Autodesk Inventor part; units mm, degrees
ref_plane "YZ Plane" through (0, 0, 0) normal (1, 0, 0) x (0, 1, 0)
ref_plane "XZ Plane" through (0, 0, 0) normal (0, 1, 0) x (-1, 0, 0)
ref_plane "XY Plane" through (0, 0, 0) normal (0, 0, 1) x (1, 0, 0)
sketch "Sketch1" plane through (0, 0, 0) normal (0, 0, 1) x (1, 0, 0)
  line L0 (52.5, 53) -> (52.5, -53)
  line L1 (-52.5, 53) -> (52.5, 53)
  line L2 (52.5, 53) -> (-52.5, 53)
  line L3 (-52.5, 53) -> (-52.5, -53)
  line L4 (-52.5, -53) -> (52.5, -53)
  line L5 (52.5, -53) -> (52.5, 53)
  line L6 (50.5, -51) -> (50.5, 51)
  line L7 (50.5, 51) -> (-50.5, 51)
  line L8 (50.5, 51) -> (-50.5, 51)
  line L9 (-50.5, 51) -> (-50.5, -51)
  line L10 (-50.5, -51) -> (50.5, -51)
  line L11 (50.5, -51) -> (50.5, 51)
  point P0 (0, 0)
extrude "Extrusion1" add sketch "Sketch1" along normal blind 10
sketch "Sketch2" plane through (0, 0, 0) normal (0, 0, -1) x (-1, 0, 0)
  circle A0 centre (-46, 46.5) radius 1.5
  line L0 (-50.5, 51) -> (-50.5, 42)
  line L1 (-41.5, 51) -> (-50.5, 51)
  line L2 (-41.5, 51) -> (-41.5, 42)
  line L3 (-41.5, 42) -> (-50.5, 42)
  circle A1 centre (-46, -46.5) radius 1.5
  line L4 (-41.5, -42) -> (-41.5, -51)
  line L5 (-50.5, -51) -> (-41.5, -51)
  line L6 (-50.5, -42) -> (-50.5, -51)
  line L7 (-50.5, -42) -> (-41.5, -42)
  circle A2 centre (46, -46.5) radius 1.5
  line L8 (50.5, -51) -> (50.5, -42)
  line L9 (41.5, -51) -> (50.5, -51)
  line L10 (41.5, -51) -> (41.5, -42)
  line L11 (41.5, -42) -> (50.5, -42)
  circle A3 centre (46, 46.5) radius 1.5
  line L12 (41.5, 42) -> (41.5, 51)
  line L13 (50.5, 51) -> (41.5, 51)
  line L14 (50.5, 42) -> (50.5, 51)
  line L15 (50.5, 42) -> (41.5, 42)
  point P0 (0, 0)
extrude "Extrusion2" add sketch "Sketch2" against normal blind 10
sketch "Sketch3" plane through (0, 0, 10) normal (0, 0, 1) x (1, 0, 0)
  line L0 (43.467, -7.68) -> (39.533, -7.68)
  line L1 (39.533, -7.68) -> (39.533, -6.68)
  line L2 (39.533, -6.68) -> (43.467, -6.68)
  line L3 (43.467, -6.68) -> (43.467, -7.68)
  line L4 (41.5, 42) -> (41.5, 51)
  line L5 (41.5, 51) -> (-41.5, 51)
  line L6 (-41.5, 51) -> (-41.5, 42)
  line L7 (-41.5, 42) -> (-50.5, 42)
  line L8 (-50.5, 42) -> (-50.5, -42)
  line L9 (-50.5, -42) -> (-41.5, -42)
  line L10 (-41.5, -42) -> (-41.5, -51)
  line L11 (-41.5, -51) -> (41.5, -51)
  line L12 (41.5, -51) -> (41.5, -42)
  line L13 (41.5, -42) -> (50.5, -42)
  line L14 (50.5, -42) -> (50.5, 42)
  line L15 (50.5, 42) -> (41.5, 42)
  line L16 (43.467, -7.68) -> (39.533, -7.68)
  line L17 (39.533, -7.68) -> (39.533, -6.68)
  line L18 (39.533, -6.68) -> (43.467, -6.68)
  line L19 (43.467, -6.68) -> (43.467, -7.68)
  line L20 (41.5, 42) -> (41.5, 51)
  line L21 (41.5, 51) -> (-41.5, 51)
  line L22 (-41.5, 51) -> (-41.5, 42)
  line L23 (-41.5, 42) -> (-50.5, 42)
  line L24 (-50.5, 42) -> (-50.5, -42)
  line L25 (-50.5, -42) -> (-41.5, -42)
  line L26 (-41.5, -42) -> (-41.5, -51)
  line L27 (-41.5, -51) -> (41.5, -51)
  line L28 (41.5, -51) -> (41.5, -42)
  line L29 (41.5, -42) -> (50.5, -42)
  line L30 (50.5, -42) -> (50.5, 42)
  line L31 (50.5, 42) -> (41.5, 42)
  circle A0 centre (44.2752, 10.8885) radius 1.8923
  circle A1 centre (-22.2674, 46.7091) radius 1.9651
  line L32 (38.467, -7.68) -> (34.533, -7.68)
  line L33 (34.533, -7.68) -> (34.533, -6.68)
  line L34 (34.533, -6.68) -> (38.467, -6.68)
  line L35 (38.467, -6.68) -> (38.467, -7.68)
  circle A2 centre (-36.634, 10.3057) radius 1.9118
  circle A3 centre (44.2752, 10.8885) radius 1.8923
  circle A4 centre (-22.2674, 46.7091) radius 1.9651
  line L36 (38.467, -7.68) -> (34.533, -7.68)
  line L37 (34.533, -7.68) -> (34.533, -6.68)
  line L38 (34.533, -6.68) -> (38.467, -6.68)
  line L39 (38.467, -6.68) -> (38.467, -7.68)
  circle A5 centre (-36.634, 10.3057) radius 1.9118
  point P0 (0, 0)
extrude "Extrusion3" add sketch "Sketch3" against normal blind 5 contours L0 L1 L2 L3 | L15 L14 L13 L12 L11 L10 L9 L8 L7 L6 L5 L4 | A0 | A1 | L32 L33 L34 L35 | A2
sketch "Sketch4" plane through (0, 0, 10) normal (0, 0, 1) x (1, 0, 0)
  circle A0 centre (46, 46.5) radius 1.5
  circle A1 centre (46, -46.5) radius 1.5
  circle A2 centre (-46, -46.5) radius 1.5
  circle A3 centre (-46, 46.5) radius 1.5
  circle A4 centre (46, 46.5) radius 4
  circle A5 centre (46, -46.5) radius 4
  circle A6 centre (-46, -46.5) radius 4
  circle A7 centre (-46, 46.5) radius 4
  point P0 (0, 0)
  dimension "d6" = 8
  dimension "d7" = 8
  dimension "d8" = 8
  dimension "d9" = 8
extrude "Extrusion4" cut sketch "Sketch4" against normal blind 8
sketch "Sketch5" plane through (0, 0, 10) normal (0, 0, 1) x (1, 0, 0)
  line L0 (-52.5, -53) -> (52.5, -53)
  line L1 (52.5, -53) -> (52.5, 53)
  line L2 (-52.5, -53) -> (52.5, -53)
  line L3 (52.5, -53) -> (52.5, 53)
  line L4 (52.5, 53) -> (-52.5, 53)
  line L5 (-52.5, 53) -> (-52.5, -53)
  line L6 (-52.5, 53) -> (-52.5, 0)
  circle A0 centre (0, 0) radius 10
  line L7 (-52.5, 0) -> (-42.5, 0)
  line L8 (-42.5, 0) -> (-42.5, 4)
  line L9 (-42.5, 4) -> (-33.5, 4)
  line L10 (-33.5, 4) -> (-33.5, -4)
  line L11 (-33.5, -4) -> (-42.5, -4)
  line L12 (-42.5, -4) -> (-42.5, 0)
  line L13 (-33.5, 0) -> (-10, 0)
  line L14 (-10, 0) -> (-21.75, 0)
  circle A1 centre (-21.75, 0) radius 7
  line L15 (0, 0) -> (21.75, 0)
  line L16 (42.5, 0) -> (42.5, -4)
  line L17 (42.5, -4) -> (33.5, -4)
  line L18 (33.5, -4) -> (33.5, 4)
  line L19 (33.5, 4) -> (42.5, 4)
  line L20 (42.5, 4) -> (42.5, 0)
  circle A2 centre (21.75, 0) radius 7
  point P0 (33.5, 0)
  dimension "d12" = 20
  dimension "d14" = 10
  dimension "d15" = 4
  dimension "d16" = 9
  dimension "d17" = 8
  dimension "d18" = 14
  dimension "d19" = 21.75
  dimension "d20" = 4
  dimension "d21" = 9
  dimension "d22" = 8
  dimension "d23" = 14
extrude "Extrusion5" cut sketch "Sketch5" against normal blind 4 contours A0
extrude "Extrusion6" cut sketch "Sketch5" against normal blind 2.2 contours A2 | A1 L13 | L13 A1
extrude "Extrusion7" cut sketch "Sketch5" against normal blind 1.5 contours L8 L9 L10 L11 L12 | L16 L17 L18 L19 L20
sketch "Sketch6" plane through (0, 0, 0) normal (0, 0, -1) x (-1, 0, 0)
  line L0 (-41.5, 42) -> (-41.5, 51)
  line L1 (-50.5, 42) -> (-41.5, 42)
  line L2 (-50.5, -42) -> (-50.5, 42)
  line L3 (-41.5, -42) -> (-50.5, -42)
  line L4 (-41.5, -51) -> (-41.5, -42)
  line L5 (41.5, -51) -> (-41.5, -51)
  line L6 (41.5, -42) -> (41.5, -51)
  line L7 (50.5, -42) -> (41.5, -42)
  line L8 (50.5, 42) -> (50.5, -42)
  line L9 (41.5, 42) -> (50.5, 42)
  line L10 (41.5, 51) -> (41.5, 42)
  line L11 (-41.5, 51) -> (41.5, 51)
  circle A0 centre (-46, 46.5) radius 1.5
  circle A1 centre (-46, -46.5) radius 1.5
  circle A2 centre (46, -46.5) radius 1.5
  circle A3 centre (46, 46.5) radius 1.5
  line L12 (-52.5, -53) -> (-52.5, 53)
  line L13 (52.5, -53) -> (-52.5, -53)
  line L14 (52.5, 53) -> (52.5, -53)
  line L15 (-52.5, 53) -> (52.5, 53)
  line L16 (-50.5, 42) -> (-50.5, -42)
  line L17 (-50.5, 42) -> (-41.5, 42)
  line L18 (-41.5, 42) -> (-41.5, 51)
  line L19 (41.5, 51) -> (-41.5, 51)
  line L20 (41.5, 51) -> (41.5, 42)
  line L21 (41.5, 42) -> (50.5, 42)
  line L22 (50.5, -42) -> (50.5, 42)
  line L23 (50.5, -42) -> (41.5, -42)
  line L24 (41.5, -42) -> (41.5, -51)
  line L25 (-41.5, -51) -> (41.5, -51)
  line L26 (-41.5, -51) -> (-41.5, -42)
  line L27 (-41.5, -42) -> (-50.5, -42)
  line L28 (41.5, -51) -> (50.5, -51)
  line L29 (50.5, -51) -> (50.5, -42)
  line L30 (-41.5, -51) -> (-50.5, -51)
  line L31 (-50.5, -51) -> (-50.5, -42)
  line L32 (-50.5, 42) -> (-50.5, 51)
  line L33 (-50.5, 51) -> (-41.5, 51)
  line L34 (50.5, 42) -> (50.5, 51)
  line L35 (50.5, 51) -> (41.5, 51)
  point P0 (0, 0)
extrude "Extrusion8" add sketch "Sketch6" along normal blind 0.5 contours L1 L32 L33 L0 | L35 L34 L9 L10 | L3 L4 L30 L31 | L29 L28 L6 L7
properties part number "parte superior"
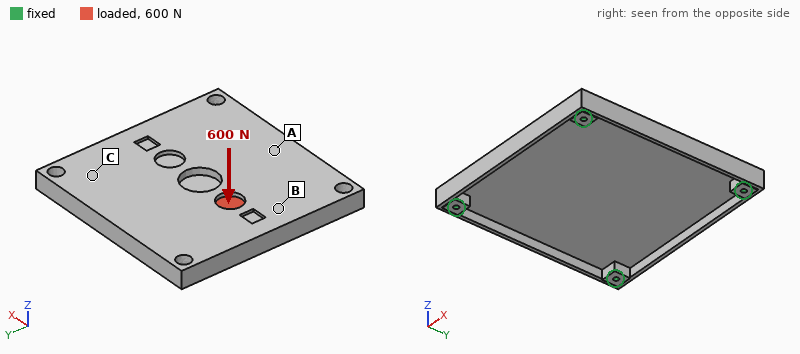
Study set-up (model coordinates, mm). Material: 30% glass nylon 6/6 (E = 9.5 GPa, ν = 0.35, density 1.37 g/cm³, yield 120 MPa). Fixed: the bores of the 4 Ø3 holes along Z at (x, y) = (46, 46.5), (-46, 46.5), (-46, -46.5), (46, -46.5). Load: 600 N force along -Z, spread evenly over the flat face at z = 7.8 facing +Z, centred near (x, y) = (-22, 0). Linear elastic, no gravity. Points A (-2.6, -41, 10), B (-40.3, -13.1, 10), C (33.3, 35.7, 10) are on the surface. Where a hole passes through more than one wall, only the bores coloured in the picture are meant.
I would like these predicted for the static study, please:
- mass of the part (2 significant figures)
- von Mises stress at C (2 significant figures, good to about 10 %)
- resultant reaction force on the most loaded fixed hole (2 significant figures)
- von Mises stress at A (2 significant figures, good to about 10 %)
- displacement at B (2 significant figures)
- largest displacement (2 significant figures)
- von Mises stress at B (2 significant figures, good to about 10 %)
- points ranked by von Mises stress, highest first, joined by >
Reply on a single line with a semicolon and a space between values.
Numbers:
79 g; 4.7 MPa; 490 N; 9.0 MPa; 0.48 mm; 0.86 mm; 18 MPa; B > A > C
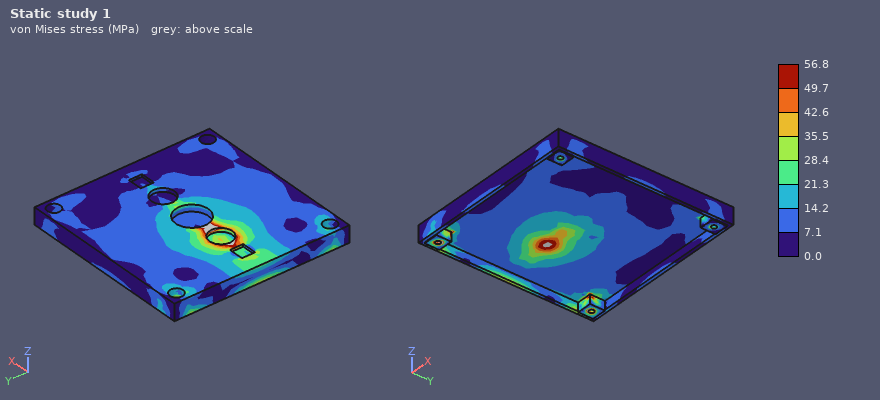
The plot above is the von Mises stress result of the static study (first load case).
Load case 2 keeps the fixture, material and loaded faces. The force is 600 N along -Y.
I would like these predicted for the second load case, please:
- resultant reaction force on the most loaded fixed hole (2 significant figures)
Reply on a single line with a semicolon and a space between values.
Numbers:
190 N
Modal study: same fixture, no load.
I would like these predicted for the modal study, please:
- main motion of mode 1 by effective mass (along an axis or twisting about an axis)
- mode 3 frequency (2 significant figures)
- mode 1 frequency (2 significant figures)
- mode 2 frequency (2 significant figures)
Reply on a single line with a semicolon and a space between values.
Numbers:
along Z; 1800 Hz; 980 Hz; 1700 Hz
